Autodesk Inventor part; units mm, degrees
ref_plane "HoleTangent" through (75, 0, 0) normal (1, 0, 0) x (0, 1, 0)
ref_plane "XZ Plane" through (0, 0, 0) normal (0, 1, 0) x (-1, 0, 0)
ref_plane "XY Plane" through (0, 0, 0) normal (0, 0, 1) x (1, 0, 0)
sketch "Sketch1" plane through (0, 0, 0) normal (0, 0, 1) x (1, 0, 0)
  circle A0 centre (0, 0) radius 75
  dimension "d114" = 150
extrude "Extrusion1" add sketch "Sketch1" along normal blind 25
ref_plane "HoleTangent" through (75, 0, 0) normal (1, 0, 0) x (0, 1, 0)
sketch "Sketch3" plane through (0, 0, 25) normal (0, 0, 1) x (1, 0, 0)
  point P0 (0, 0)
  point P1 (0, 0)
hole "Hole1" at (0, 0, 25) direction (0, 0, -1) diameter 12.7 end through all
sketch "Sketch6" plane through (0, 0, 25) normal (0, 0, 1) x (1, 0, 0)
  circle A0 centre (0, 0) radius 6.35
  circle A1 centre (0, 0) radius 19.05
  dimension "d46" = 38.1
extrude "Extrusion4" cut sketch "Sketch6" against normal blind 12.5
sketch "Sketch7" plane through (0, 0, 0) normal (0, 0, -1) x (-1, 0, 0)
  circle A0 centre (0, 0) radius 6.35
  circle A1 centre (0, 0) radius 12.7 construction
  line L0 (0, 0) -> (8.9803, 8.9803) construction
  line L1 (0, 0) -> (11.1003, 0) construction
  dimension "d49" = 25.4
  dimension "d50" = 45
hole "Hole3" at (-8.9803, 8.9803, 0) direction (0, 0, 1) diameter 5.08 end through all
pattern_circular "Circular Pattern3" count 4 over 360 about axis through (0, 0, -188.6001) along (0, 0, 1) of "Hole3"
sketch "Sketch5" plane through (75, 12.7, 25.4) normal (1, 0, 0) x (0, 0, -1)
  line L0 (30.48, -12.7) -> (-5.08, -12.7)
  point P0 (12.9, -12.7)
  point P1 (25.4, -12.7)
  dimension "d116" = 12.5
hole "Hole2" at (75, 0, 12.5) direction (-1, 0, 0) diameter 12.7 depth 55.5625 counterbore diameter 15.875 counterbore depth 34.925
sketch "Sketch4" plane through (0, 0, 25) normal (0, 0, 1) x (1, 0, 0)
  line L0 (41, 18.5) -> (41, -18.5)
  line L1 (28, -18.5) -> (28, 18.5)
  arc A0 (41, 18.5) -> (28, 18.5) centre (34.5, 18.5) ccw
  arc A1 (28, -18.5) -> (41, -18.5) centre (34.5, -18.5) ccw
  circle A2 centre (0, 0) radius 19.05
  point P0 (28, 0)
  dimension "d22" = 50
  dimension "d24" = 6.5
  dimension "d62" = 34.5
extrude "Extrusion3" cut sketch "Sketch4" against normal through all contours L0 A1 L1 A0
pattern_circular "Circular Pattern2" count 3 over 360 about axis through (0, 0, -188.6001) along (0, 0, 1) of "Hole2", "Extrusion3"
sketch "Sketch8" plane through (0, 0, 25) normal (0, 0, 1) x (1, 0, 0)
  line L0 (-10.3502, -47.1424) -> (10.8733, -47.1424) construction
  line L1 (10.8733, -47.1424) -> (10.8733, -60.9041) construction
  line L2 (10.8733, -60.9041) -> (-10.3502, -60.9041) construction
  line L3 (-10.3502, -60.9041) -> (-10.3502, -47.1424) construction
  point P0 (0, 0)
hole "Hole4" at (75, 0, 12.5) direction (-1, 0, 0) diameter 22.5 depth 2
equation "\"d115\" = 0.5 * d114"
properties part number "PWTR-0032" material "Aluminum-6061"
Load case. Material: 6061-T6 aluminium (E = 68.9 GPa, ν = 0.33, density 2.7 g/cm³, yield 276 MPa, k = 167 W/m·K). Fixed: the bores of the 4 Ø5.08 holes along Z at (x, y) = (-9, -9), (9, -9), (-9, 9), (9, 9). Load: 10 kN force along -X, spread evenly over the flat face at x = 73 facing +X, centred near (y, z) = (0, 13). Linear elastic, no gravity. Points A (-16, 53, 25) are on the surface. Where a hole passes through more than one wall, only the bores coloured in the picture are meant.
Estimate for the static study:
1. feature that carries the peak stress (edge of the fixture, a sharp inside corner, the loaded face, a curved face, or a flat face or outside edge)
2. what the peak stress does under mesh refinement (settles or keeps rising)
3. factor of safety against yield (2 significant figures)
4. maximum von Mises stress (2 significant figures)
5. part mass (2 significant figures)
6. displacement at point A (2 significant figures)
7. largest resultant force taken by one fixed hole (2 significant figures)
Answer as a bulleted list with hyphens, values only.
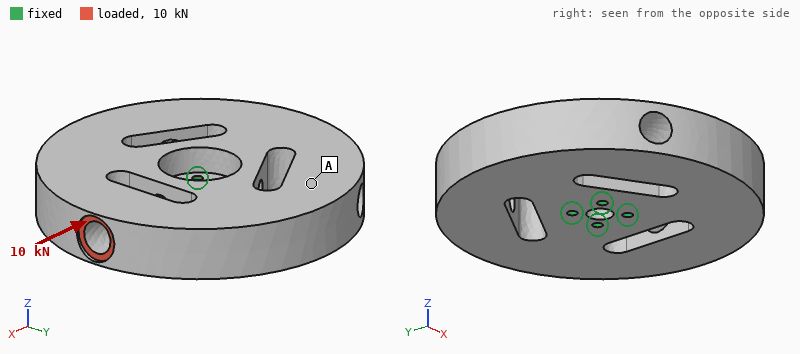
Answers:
- the loaded face
- settles
- 2.8
- 100 MPa
- 960 g
- 15 µm
- 3.0 kN
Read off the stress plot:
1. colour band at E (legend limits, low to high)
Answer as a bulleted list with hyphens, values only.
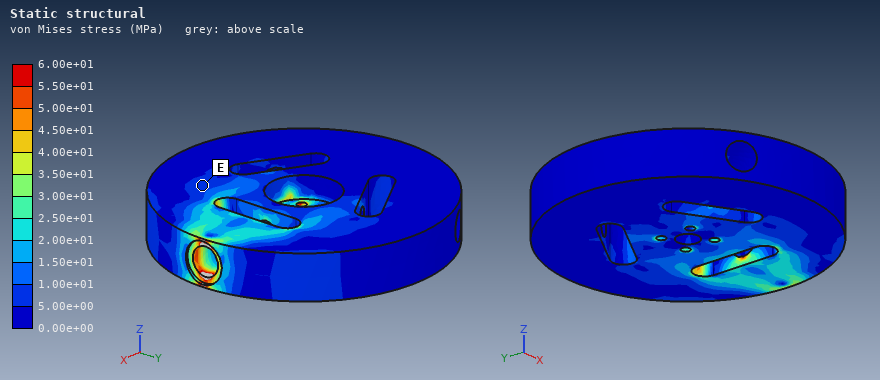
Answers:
- 5.00e+00 to 1.00e+01 MPa
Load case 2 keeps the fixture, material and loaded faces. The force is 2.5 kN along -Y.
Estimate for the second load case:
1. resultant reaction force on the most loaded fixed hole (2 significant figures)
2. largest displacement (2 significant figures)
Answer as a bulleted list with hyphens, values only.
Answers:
- 3.6 kN
- 30 µm
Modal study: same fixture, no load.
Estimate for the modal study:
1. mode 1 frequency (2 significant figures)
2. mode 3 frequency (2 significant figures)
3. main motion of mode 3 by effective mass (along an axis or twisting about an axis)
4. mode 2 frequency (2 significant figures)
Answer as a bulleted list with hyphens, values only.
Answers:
- 1700 Hz
- 2300 Hz
- twisting about Z
- 1700 Hz
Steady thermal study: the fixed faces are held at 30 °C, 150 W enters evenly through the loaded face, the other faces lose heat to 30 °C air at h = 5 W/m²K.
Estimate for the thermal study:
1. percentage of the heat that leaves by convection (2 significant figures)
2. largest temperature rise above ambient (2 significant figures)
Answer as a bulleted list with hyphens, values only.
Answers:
- 3.6 %
- 74 K
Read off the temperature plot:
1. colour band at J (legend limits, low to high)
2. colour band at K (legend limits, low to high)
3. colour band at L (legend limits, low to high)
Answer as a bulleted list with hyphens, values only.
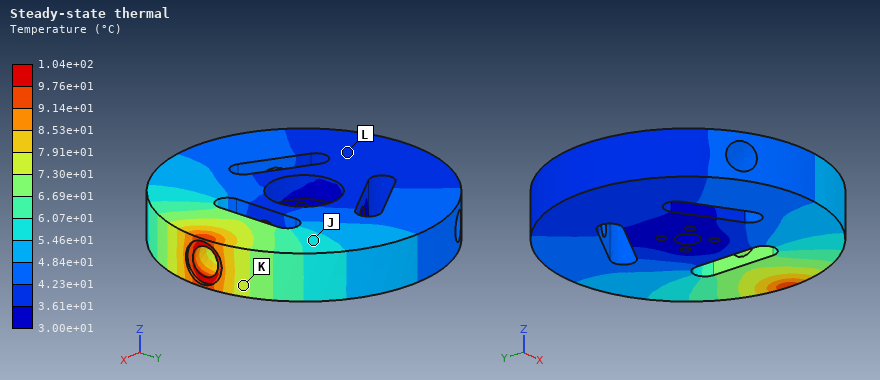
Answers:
- 5.46e+01 to 6.07e+01 °C
- 7.30e+01 to 7.91e+01 °C
- 3.61e+01 to 4.23e+01 °C
